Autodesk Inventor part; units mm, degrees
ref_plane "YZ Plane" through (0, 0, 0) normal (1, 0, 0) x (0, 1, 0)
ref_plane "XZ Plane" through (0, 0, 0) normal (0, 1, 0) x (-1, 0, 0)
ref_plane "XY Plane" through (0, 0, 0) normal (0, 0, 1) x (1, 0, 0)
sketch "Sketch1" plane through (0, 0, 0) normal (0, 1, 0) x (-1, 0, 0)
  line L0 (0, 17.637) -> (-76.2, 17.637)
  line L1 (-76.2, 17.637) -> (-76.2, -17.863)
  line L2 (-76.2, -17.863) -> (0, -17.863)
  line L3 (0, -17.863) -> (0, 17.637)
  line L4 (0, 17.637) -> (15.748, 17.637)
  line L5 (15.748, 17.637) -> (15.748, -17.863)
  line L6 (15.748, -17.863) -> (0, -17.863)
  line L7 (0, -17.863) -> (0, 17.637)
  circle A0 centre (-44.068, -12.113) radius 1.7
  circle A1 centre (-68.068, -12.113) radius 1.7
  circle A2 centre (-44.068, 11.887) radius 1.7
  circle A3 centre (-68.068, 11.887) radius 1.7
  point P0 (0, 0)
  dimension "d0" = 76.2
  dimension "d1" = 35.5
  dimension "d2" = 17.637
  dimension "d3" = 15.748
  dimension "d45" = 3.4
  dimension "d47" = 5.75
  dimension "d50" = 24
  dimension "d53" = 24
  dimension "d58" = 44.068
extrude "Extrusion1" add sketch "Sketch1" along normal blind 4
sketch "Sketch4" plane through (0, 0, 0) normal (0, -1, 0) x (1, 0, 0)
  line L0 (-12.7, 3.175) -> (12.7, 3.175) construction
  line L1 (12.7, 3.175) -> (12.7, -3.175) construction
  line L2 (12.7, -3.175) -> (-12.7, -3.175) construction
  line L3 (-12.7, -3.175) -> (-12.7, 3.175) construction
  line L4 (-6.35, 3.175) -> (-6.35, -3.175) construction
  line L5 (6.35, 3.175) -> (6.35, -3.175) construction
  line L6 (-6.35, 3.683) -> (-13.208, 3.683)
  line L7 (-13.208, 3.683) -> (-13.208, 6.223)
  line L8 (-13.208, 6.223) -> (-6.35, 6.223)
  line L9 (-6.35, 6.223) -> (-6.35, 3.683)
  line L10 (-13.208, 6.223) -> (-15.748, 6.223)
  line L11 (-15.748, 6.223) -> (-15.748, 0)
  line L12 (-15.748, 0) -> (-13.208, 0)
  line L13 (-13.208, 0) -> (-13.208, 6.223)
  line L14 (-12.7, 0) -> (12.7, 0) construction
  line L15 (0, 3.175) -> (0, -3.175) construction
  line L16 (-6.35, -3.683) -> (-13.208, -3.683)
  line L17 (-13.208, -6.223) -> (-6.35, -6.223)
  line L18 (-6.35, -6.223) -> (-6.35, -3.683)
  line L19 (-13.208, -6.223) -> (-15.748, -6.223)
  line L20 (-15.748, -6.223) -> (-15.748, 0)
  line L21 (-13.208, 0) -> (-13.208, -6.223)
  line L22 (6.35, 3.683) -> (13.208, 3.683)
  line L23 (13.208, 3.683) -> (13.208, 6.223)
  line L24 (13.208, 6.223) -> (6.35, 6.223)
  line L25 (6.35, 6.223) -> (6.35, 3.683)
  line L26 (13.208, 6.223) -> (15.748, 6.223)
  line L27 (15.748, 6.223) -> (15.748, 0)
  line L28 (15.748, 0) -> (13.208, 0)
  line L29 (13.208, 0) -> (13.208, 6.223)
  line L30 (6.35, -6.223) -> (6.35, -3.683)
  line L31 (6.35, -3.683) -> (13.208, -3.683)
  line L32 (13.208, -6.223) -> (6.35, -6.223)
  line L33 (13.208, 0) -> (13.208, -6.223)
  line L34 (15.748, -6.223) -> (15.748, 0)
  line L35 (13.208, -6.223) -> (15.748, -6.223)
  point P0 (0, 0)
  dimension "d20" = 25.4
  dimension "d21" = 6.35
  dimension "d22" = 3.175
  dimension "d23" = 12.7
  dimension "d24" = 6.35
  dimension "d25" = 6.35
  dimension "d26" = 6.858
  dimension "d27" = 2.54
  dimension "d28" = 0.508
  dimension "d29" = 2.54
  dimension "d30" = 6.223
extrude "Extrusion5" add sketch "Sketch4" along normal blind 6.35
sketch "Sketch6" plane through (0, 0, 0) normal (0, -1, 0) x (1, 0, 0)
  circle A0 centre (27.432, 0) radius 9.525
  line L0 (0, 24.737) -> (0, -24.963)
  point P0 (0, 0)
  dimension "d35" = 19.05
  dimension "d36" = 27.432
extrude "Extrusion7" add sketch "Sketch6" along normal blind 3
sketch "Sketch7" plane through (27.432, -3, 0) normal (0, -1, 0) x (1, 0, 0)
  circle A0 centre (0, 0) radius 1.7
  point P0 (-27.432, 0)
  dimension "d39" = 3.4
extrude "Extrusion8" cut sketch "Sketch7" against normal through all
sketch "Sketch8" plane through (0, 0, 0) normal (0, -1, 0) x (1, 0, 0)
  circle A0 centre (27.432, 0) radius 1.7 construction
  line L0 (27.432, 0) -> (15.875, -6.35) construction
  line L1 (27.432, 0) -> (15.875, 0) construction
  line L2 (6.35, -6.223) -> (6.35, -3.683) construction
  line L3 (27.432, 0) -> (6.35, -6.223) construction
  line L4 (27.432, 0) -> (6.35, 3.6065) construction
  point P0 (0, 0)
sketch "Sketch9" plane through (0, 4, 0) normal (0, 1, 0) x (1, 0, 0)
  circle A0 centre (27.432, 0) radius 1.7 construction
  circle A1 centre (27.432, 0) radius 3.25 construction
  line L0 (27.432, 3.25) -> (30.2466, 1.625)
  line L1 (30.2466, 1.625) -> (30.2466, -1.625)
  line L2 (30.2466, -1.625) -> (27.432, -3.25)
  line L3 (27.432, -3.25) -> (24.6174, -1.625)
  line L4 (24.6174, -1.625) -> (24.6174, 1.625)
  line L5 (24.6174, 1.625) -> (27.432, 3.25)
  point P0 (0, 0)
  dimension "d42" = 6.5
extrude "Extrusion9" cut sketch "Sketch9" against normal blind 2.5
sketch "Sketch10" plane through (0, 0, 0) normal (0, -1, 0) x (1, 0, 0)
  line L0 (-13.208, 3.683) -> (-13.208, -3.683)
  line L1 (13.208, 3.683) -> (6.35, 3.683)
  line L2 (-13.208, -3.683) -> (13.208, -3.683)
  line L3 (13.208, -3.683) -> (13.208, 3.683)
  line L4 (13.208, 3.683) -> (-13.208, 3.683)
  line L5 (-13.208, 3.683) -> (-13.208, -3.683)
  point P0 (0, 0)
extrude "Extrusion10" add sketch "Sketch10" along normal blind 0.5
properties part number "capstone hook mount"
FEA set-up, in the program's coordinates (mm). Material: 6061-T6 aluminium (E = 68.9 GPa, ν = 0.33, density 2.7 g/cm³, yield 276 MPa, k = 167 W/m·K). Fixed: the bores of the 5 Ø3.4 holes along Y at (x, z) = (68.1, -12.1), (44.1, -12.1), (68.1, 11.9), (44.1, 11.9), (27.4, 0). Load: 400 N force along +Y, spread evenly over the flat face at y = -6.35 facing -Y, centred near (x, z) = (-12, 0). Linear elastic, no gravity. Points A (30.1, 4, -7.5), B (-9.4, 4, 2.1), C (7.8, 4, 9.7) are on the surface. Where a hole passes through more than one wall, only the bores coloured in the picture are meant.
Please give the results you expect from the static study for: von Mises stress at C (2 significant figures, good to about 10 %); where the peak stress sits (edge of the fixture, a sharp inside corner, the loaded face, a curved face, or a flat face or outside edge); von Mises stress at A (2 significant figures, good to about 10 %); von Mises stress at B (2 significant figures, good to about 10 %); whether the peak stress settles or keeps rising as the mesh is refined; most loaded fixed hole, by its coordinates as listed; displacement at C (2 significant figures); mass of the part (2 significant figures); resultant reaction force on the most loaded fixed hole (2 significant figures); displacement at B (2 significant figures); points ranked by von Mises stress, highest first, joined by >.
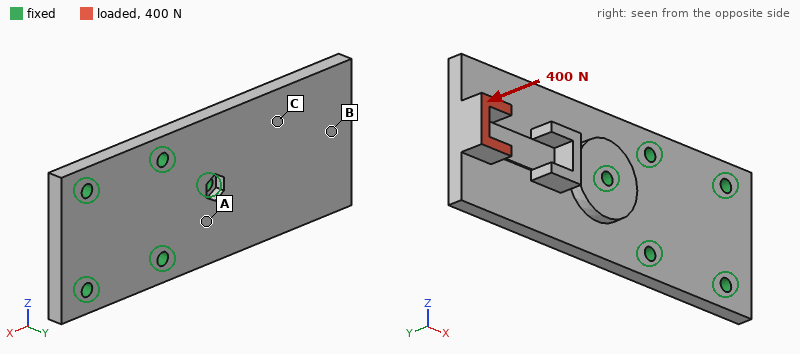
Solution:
66 MPa
edge of the fixture
43 MPa
16 MPa
keeps rising
(27.4, 0)
0.13 mm
39 g
1.4 kN
0.40 mm
C > A > B
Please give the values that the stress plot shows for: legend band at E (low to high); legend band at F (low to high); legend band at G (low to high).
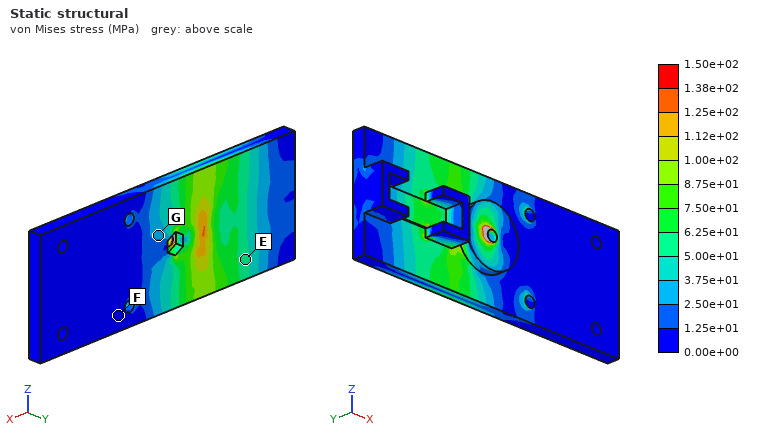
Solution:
5.00e+01 to 6.25e+01 MPa
0.00e+00 to 1.25e+01 MPa
2.50e+01 to 3.75e+01 MPa
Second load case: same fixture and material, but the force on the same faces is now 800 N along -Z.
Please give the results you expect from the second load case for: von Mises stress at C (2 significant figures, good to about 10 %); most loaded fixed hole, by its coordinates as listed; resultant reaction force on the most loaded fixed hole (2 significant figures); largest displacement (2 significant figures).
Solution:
39 MPa
(27.4, 0)
1.4 kN
0.19 mm
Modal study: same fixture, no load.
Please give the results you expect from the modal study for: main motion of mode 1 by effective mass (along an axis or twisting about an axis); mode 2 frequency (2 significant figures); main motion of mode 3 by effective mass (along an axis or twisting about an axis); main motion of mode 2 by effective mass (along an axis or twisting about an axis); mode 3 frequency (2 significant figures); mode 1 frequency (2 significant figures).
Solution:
along Y
4400 Hz
along Z
twisting about X
7300 Hz
1900 Hz
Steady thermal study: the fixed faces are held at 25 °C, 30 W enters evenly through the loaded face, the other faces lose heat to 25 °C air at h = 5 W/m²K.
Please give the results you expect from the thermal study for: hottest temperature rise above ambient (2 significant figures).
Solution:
72 K
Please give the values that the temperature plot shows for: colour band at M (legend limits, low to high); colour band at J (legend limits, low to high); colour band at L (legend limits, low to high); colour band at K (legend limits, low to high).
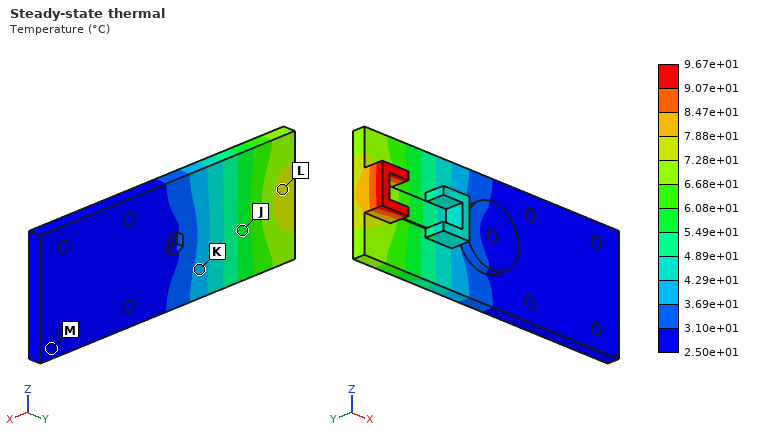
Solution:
2.50e+01 to 3.10e+01 °C
5.49e+01 to 6.08e+01 °C
7.28e+01 to 7.88e+01 °C
3.69e+01 to 4.29e+01 °C
